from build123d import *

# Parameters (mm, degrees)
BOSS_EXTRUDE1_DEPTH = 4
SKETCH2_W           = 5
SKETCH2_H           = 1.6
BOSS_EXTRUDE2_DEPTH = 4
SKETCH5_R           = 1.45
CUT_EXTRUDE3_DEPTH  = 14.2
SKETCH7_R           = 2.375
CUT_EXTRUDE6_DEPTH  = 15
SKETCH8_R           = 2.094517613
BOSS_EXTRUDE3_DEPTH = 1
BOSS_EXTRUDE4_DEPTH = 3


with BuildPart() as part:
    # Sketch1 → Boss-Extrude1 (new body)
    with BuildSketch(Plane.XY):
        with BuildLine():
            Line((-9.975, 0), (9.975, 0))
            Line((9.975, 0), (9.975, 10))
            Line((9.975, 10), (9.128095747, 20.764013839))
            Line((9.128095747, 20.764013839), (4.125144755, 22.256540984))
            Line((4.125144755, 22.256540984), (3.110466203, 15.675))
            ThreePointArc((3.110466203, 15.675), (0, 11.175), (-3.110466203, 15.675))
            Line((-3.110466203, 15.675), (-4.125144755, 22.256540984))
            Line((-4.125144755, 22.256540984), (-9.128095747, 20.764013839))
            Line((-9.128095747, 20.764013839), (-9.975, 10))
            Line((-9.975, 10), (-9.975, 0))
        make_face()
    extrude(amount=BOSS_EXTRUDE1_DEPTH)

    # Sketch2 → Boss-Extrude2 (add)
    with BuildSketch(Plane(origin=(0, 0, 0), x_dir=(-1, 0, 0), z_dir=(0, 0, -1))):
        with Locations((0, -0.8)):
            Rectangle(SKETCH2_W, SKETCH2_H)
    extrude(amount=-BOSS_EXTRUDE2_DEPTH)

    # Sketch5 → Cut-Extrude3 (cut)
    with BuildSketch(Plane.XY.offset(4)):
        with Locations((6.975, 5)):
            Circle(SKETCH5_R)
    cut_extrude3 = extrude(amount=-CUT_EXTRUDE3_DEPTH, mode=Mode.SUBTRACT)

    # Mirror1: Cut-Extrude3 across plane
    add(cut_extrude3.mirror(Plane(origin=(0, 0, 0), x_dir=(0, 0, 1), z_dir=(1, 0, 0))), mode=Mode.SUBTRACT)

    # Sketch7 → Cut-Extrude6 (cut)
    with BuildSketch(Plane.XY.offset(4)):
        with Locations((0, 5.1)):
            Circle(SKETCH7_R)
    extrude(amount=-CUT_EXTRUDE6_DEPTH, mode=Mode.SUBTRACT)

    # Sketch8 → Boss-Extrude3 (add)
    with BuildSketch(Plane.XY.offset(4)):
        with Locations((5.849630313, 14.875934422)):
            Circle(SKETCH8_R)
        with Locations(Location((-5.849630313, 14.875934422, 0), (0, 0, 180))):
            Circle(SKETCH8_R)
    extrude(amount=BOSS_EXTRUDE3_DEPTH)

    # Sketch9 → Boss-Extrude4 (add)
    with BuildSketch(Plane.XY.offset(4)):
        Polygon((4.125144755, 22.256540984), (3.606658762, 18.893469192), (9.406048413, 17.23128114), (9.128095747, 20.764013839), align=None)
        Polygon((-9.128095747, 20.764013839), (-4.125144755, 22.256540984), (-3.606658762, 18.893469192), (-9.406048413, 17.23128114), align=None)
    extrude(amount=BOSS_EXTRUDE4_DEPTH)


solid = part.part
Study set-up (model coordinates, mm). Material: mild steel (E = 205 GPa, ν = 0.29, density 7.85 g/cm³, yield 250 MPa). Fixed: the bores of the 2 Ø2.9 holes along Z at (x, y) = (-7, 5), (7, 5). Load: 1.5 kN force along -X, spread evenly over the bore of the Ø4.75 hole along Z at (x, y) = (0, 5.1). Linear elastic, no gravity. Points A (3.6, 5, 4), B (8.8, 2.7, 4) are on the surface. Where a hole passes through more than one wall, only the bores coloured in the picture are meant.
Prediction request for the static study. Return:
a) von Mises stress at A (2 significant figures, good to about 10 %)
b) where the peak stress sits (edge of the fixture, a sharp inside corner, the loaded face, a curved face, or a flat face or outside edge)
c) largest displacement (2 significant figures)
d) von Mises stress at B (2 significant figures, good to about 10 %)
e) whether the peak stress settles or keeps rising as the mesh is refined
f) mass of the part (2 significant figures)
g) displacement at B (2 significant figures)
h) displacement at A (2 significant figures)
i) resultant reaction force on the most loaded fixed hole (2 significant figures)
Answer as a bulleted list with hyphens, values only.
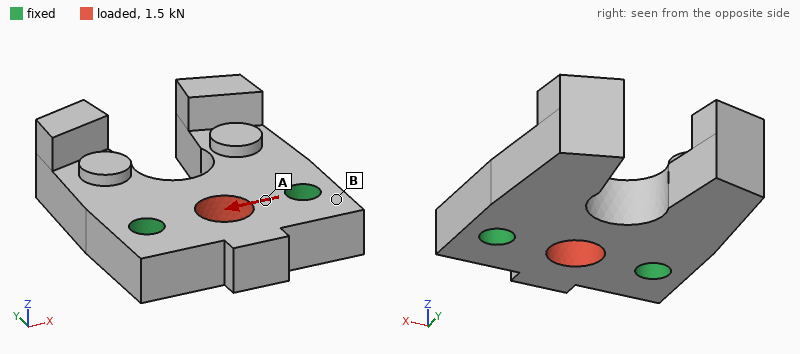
- 33 MPa
- edge of the fixture
- 0.89 µm
- 8.8 MPa
- keeps rising
- 11 g
- 0.15 µm
- 0.35 µm
- 750 N
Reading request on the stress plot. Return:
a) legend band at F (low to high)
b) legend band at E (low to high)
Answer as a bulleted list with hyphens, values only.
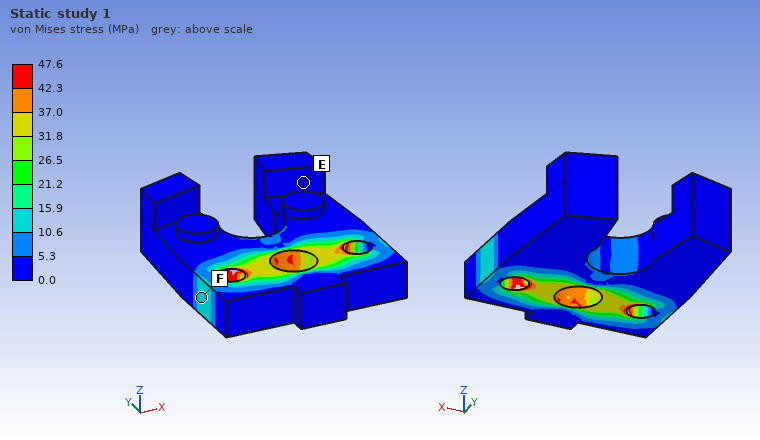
- 10.6 to 15.9 MPa
- 0.0 to 5.3 MPa
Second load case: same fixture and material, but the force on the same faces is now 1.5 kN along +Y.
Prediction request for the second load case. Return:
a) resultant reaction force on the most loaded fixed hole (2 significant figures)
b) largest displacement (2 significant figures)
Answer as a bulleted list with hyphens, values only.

- 750 N
- 2.5 µm
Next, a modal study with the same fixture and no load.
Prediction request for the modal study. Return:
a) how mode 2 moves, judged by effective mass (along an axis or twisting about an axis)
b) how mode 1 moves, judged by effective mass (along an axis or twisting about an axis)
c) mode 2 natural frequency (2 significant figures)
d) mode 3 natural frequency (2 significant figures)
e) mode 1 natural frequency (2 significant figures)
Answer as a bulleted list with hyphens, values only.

- twisting about Y
- along Z
- 13 kHz
- 24 kHz
- 12 kHz
